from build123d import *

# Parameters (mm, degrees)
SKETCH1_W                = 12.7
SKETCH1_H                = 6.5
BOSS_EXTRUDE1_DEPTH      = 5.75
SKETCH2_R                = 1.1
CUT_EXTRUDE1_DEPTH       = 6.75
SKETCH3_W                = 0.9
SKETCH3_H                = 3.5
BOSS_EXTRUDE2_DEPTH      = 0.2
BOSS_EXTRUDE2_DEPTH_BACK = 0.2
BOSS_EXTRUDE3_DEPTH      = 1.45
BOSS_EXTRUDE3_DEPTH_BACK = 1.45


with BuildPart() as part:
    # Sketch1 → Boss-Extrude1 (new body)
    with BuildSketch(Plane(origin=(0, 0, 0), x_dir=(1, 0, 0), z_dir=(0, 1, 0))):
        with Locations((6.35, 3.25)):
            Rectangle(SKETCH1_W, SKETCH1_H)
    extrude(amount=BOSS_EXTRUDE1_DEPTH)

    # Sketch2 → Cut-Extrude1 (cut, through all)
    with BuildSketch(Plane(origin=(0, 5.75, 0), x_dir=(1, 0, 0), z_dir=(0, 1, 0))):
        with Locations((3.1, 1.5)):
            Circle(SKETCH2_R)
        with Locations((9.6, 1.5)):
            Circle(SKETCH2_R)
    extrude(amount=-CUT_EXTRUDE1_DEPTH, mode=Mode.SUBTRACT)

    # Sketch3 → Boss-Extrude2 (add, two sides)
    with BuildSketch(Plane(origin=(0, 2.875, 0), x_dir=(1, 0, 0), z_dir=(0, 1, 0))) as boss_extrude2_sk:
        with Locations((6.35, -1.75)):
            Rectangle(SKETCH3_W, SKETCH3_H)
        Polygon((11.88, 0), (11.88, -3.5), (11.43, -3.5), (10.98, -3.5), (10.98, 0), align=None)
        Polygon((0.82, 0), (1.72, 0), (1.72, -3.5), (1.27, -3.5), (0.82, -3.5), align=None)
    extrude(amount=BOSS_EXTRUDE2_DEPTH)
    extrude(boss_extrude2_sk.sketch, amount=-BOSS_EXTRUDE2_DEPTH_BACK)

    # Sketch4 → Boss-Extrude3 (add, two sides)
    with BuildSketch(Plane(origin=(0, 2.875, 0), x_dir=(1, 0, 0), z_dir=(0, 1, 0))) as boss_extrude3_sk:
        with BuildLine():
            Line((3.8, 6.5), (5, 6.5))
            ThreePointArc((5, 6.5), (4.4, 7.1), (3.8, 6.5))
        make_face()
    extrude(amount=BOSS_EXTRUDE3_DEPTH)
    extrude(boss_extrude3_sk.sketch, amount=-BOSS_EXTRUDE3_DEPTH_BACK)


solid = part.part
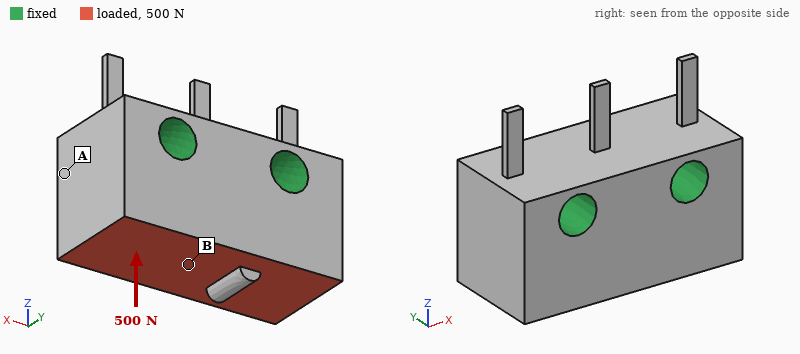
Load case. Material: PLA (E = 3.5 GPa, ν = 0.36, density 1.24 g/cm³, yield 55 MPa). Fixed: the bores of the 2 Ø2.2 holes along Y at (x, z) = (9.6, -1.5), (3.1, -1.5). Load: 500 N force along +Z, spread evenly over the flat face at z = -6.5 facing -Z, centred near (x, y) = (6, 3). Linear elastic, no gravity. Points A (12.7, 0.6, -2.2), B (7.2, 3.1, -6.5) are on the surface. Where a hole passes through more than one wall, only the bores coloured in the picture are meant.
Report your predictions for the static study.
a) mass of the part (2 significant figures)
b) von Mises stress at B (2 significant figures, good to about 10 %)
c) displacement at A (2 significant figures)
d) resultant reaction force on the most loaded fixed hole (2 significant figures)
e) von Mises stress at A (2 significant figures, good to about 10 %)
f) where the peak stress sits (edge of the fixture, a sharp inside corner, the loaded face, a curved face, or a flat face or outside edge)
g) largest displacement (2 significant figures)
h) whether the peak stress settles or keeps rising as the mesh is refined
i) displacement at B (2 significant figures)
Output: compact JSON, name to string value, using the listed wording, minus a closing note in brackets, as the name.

{"mass of the part": "0.54 g", "von Mises stress at B": "7.3 MPa", "displacement at A": "7.3 µm", "resultant reaction force on the most loaded fixed hole": "260 N", "von Mises stress at A": "2.5 MPa", "where the peak stress sits": "edge of the fixture", "largest displacement": "15 µm", "whether the peak stress settles or keeps rising as the mesh is refined": "keeps rising", "displacement at B": "9.6 µm"}
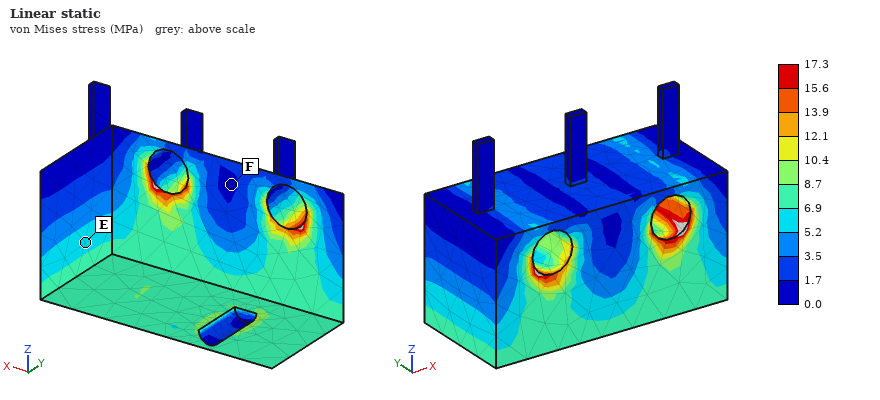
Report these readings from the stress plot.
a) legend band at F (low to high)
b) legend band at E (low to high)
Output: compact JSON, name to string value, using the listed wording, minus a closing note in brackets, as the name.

{"legend band at F": "0.0 to 1.7 MPa", "legend band at E": "5.2 to 6.9 MPa"}
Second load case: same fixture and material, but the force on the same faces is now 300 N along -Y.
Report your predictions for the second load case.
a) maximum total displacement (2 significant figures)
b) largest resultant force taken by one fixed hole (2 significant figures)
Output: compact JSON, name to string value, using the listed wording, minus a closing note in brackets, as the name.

{"maximum total displacement": "40 µm", "largest resultant force taken by one fixed hole": "150 N"}
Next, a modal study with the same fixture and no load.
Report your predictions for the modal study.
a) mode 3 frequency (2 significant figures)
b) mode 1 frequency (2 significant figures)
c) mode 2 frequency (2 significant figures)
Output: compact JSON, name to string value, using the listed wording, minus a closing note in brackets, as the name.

{"mode 3 frequency": "8500 Hz", "mode 1 frequency": "8500 Hz", "mode 2 frequency": "8500 Hz"}
